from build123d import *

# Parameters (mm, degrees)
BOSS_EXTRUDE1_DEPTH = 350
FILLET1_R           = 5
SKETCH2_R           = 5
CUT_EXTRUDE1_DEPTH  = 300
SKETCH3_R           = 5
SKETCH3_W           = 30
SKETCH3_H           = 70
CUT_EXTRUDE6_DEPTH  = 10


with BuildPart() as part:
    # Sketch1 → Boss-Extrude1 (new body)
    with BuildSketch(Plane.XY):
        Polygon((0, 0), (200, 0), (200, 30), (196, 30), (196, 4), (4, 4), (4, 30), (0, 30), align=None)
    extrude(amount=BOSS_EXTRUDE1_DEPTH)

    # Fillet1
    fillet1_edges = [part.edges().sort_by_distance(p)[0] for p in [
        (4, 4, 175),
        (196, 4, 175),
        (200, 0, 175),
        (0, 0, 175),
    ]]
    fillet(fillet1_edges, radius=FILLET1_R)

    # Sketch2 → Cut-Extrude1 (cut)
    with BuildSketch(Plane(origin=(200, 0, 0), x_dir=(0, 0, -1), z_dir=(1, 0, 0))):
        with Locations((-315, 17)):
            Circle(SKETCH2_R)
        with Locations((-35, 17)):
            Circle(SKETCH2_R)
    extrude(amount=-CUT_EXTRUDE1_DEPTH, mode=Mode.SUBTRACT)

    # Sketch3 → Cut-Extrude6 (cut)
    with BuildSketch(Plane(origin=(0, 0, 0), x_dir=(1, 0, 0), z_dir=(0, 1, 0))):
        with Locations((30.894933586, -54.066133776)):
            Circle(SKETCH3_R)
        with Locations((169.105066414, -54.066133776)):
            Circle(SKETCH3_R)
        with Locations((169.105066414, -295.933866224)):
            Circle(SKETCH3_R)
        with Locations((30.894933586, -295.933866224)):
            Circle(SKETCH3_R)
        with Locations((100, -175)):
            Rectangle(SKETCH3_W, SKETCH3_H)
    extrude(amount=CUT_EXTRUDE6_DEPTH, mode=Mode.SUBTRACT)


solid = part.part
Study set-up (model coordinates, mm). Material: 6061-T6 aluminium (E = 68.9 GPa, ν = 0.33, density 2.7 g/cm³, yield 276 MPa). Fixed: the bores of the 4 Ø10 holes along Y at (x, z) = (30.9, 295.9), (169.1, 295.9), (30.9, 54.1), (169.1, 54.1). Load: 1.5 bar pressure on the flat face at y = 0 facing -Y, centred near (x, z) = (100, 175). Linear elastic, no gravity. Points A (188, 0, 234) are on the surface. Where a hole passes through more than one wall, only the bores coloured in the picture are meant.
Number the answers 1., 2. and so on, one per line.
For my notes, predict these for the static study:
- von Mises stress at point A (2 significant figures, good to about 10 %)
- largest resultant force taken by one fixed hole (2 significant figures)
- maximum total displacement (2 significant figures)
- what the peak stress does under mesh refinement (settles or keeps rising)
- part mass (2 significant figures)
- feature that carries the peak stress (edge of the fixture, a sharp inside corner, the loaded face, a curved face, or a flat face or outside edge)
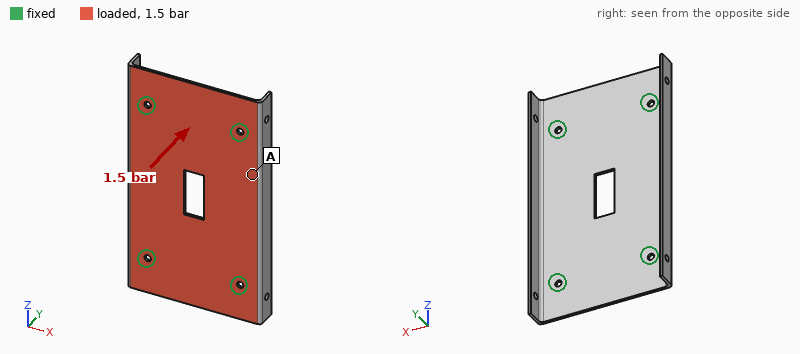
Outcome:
1. 55 MPa
2. 2.7 kN
3. 2.7 mm
4. keeps rising
5. 920 g
6. edge of the fixture
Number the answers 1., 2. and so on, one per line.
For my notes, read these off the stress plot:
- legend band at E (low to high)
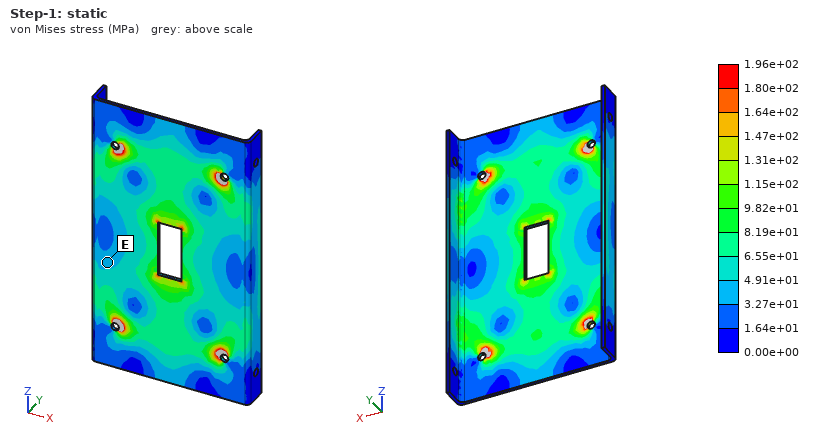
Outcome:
1. 3.27e+01 to 4.91e+01 MPa
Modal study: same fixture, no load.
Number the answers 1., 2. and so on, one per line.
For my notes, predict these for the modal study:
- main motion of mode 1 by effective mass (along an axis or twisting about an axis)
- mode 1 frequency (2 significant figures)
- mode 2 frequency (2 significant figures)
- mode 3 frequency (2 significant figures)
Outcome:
1. along Y
2. 480 Hz
3. 800 Hz
4. 850 Hz
